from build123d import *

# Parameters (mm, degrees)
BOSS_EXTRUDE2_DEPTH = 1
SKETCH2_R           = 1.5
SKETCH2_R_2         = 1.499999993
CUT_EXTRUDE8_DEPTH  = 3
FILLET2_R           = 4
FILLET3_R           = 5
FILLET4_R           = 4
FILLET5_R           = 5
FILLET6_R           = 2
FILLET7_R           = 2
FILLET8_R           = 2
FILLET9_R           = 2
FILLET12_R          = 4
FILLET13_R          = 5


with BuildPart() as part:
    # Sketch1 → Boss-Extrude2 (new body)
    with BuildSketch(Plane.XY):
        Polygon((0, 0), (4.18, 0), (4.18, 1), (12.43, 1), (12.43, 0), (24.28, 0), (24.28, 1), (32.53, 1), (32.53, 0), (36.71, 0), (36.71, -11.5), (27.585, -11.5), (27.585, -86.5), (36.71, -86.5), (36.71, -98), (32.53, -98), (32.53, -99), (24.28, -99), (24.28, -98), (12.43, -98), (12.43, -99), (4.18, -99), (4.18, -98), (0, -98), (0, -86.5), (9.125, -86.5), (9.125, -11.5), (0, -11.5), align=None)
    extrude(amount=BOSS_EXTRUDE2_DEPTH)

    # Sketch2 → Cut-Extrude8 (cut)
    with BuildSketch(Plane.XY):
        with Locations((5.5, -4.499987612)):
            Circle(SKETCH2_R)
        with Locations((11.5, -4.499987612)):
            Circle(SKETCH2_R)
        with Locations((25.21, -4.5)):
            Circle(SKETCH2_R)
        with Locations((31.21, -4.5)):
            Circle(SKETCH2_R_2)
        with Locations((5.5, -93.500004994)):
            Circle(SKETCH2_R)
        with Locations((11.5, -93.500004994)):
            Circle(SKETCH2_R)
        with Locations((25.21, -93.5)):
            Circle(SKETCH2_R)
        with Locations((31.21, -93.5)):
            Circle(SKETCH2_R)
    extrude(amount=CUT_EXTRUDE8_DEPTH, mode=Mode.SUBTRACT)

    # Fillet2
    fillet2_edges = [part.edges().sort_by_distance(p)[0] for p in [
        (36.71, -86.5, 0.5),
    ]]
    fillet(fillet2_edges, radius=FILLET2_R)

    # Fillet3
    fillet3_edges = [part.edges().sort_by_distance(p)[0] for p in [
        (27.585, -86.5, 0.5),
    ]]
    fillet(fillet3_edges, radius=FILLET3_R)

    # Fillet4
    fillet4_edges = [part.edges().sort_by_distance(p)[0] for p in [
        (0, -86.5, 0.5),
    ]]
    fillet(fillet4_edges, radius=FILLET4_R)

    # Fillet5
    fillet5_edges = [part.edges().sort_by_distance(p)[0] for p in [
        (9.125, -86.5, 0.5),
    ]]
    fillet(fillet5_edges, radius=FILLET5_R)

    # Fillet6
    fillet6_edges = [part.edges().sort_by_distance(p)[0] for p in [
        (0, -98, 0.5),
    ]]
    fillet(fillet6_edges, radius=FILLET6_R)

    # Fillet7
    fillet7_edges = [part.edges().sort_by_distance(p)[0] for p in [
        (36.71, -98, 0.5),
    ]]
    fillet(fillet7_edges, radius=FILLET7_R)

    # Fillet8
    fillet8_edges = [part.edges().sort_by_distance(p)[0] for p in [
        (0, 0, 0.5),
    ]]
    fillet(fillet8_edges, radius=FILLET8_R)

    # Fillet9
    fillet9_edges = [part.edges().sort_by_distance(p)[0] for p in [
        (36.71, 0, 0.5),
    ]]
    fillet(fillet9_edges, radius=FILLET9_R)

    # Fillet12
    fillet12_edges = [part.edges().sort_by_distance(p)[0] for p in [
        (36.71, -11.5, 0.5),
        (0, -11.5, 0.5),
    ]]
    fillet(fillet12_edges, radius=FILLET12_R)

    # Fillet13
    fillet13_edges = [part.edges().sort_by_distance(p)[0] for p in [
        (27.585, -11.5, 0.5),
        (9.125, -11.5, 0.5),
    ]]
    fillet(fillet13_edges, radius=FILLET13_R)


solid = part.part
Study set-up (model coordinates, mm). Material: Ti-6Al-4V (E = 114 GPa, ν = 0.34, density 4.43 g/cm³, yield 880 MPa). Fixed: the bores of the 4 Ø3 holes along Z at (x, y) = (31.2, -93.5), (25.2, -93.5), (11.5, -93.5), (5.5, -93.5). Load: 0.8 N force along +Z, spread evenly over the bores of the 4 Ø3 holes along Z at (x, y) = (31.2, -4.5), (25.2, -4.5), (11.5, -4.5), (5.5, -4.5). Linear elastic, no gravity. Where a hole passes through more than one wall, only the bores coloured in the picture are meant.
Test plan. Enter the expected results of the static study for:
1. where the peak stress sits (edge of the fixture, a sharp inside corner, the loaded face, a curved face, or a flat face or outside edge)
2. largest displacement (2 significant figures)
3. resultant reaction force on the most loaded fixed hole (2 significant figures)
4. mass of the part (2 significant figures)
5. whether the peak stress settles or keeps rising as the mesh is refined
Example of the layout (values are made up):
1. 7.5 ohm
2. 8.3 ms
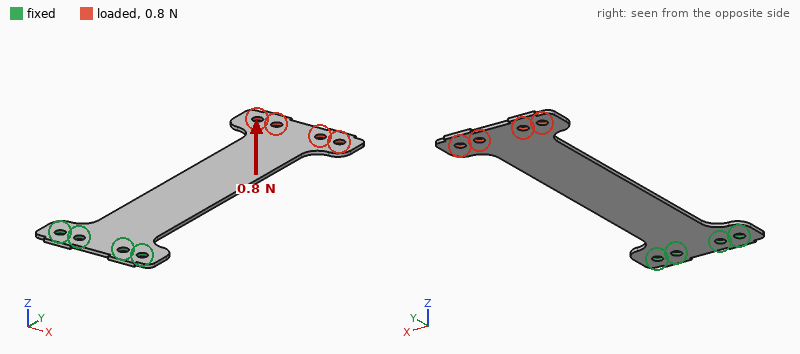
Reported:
1. edge of the fixture
2. 1.0 mm
3. 1.1 N
4. 9.8 g
5. keeps rising
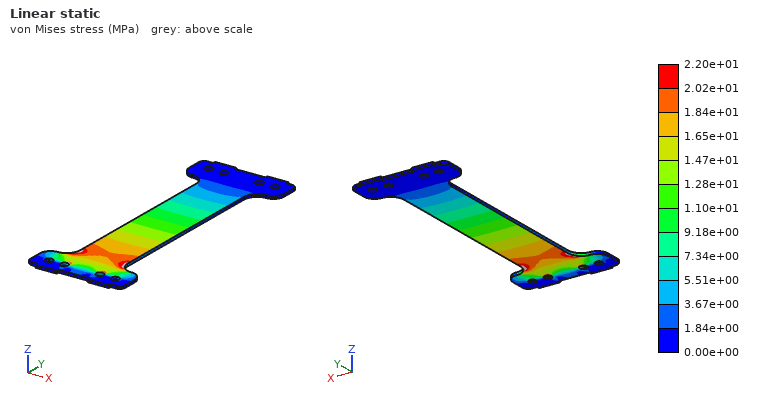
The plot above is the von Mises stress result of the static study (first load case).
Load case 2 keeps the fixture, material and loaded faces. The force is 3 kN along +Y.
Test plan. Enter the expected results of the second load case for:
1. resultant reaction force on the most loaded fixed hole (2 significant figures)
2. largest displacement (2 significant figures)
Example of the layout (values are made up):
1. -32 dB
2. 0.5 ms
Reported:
1. 1.1 kN
2. 0.14 mm
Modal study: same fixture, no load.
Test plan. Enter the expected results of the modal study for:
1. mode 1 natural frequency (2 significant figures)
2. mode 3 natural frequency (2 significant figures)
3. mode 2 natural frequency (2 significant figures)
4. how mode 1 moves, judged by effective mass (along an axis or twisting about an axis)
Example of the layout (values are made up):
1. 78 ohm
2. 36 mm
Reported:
1. 85 Hz
2. 580 Hz
3. 570 Hz
4. along Z
